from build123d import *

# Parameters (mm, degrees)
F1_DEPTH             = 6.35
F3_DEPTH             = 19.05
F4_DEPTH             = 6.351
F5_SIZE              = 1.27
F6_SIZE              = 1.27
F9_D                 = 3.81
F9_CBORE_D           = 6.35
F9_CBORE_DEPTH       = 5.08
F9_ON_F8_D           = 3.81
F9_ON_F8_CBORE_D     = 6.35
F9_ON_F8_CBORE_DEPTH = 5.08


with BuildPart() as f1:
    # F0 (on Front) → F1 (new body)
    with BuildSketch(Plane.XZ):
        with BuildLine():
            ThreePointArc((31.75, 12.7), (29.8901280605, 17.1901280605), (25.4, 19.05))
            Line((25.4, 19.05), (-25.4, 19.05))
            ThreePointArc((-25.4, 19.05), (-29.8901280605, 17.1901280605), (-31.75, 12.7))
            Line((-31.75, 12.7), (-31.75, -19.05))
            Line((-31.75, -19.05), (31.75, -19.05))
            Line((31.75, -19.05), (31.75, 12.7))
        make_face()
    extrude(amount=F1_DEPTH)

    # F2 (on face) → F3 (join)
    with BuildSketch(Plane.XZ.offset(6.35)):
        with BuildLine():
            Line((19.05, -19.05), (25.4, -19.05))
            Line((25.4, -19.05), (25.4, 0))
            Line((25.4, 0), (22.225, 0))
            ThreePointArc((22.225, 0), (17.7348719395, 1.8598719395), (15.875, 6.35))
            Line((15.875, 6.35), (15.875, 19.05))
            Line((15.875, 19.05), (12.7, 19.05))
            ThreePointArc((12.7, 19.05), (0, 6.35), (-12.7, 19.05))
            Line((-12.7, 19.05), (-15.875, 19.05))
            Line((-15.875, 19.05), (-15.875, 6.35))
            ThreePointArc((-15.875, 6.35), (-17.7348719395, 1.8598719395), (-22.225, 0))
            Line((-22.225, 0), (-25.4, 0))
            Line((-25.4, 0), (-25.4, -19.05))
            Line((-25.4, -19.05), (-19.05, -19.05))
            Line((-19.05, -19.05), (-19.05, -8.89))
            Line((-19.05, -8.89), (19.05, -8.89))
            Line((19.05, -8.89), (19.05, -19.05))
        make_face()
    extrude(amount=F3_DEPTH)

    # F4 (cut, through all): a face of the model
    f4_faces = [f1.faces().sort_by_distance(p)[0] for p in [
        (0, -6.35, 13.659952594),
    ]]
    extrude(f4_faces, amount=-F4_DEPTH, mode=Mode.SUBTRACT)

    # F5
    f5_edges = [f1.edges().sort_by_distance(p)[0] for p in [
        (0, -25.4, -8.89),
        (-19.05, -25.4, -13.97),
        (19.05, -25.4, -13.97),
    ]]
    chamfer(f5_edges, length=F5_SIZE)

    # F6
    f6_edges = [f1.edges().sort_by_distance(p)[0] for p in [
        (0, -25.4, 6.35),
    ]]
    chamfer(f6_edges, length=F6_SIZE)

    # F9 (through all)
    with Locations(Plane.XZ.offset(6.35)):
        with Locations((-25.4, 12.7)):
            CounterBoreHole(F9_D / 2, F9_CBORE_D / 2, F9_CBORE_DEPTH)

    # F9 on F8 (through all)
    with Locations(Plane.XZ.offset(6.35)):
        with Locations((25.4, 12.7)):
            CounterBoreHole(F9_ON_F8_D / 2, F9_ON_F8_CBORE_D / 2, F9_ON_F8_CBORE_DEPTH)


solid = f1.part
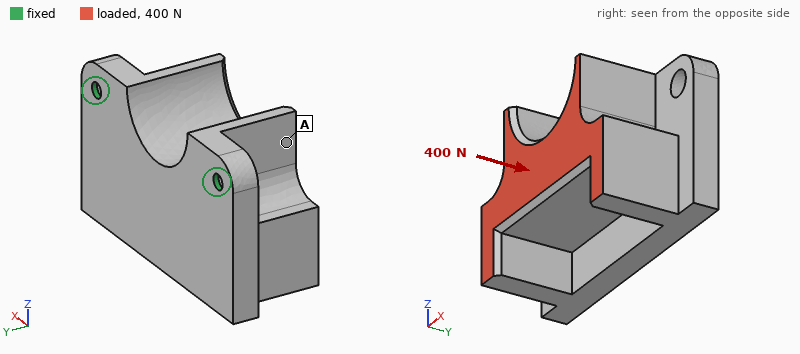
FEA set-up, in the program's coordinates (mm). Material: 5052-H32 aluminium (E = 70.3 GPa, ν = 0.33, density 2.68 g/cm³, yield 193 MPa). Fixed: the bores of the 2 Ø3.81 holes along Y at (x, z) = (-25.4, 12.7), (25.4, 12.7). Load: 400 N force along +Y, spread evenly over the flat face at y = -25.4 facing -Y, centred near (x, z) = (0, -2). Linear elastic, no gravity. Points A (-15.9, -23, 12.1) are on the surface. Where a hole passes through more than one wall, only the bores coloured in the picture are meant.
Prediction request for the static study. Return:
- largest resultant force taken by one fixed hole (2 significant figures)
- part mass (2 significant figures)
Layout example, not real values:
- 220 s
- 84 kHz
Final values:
- 200 N
- 84 g
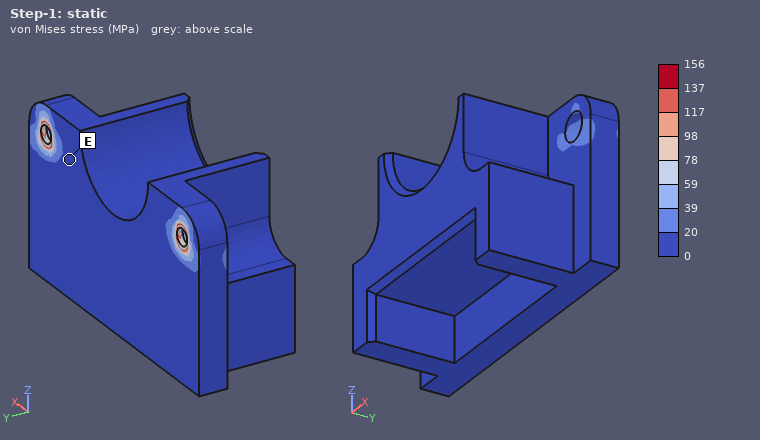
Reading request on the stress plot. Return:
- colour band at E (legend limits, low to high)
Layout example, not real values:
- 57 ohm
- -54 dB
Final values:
- 0 to 20 MPa
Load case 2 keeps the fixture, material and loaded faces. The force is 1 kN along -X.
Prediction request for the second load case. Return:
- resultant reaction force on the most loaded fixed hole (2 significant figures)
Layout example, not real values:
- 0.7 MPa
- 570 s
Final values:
- 760 N
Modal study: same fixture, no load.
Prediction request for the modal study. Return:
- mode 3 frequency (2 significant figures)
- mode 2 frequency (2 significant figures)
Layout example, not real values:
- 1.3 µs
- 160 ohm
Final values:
- 7700 Hz
- 6100 Hz
